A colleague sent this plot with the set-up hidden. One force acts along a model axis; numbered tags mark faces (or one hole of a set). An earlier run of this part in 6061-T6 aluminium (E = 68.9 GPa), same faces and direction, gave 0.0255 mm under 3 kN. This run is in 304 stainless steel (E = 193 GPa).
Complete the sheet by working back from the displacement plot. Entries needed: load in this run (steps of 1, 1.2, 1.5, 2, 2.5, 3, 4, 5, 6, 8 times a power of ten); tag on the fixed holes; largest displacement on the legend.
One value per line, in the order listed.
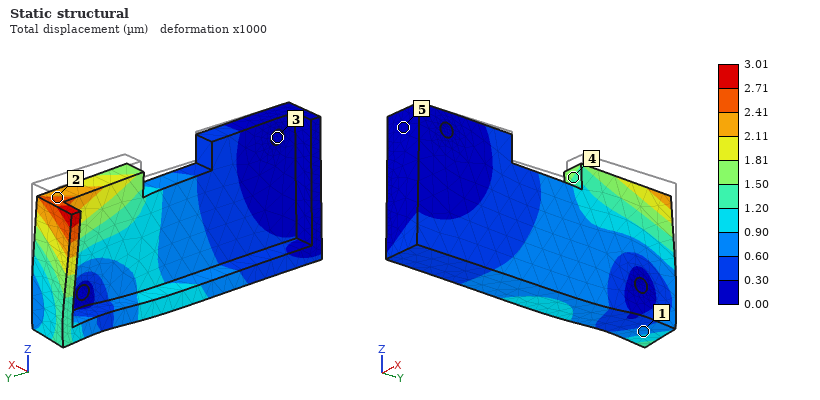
1 kN
3
3.01 µm
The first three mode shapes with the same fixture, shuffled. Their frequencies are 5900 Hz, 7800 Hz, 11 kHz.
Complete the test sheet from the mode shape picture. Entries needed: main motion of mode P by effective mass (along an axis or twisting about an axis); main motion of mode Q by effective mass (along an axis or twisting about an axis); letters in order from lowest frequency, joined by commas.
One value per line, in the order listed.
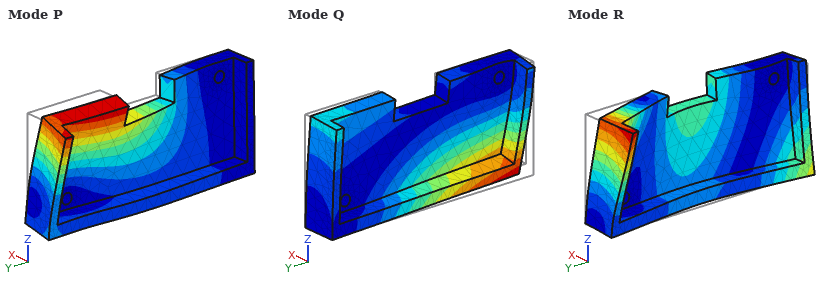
along X
along X
Q, P, R
